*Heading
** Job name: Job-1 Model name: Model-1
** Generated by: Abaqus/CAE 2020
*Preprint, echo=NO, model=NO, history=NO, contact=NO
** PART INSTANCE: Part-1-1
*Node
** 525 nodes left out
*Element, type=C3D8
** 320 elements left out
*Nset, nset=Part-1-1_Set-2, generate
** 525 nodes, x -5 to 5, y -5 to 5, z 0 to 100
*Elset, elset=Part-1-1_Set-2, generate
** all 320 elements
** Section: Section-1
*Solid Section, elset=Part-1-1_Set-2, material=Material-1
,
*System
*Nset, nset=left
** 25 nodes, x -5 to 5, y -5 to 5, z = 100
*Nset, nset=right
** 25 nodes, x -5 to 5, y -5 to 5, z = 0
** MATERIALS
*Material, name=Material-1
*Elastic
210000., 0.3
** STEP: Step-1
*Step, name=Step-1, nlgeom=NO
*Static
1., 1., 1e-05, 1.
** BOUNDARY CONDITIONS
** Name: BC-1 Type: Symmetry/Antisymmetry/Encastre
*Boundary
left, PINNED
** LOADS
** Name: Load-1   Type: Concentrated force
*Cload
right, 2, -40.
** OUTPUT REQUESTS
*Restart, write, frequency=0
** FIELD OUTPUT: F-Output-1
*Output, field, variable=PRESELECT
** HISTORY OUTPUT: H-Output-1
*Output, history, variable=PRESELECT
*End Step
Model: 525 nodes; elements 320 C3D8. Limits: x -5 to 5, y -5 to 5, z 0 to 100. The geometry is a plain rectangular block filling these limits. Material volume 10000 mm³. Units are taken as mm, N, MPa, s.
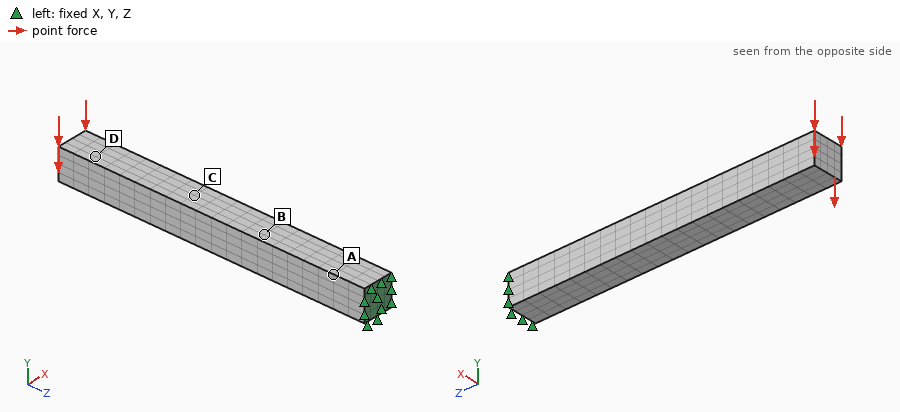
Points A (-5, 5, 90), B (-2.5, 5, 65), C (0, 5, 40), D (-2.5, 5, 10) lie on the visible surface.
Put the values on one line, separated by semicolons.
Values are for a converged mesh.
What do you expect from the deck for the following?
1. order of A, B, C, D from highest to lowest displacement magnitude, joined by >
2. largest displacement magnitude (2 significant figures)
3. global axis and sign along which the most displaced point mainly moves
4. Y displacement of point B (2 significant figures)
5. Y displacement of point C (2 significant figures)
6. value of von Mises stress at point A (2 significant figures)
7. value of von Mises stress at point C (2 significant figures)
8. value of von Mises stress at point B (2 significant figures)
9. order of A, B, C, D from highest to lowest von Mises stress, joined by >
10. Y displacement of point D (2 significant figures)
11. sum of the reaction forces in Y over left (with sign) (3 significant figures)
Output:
D > C > B > A; 1.9 mm; -Y; -0.31 mm; -0.82 mm; 530 MPa; 240 MPa; 390 MPa; A > B > C > D; -1.6 mm; 1000 N
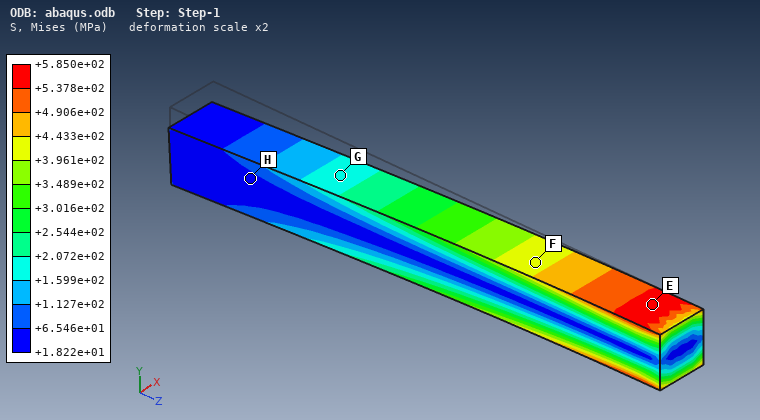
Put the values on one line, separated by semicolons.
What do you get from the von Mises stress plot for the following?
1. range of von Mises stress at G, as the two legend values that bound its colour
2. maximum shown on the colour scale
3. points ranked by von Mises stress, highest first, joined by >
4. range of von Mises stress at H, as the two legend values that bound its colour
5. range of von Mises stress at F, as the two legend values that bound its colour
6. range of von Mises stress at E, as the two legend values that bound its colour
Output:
+1.599e+02 to +2.072e+02 MPa; +5.850e+02 MPa; E > F > G > H; +1.822e+01 to +6.546e+01 MPa; +3.961e+02 to +4.433e+02 MPa; +5.378e+02 to +5.850e+02 MPa
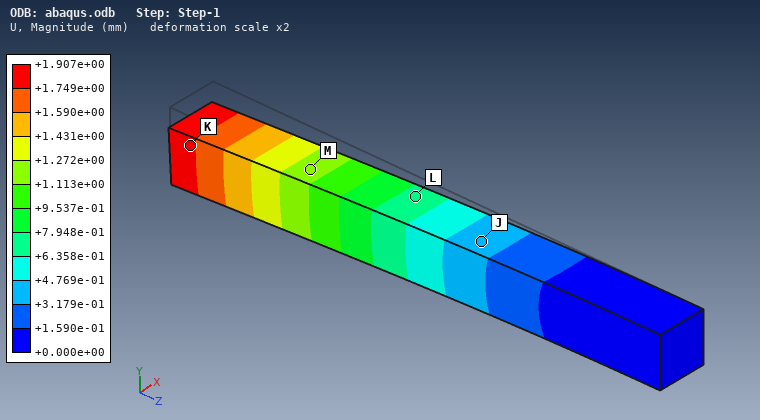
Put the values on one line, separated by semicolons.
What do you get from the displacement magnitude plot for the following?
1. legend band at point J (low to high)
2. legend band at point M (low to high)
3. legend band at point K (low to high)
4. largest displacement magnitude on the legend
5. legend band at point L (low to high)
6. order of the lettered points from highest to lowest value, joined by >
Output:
+3.179e-01 to +4.769e-01 mm; +1.113e+00 to +1.272e+00 mm; +1.749e+00 to +1.907e+00 mm; +1.907e+00 mm; +6.358e-01 to +7.948e-01 mm; K > M > L > J
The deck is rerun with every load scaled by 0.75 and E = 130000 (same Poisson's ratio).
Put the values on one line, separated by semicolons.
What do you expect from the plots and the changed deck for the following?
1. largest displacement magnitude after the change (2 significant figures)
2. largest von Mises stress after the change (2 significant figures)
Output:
2.3 mm; 440 MPa
